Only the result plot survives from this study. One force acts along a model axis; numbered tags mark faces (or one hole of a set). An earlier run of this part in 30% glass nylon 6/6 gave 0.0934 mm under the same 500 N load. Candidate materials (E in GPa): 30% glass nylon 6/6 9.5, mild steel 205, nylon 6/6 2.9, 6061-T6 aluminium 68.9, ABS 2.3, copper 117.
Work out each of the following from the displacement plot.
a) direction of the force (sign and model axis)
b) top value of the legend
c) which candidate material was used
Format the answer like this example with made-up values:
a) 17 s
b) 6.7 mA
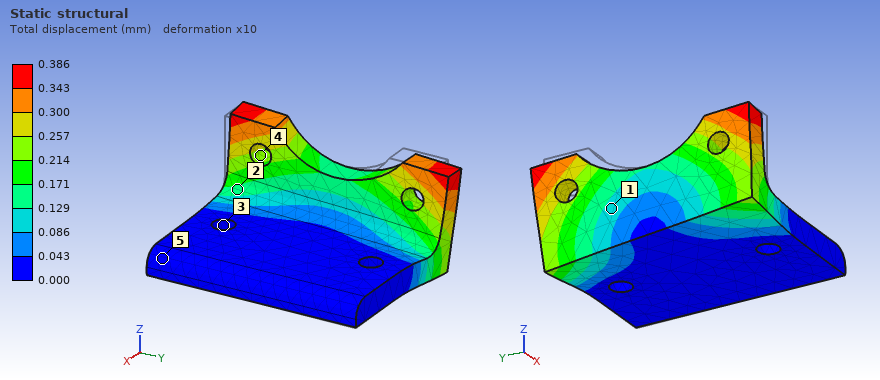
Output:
a) +Y
b) 0.386 mm
c) ABS
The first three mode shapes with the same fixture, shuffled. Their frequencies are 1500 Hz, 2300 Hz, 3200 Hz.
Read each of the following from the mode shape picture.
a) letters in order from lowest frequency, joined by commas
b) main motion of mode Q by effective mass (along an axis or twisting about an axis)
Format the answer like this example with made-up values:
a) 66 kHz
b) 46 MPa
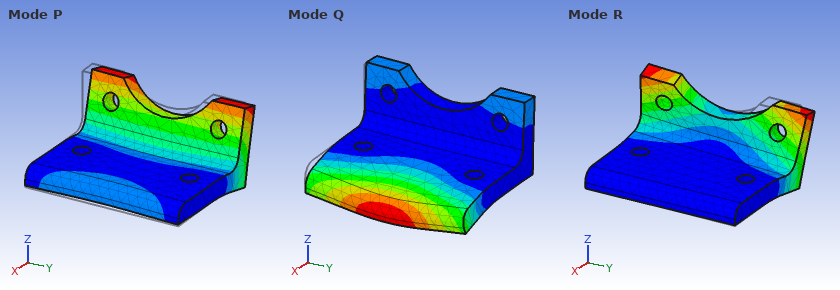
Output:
a) P, R, Q
b) along Z
